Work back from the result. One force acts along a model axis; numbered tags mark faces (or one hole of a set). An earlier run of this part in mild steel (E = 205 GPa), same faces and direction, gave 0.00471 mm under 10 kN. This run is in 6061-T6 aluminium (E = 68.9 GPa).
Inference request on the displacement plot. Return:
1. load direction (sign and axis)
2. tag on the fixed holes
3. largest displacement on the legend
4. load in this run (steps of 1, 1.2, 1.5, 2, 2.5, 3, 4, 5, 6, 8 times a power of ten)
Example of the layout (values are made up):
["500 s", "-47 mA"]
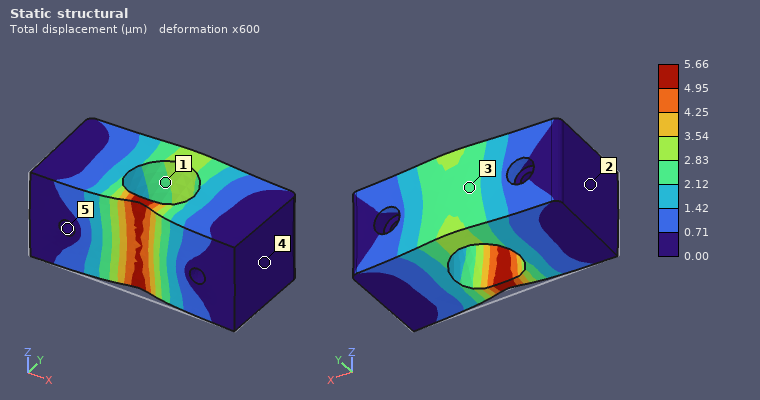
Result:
["+Y", "5", "5.66 µm", "4 kN"]
